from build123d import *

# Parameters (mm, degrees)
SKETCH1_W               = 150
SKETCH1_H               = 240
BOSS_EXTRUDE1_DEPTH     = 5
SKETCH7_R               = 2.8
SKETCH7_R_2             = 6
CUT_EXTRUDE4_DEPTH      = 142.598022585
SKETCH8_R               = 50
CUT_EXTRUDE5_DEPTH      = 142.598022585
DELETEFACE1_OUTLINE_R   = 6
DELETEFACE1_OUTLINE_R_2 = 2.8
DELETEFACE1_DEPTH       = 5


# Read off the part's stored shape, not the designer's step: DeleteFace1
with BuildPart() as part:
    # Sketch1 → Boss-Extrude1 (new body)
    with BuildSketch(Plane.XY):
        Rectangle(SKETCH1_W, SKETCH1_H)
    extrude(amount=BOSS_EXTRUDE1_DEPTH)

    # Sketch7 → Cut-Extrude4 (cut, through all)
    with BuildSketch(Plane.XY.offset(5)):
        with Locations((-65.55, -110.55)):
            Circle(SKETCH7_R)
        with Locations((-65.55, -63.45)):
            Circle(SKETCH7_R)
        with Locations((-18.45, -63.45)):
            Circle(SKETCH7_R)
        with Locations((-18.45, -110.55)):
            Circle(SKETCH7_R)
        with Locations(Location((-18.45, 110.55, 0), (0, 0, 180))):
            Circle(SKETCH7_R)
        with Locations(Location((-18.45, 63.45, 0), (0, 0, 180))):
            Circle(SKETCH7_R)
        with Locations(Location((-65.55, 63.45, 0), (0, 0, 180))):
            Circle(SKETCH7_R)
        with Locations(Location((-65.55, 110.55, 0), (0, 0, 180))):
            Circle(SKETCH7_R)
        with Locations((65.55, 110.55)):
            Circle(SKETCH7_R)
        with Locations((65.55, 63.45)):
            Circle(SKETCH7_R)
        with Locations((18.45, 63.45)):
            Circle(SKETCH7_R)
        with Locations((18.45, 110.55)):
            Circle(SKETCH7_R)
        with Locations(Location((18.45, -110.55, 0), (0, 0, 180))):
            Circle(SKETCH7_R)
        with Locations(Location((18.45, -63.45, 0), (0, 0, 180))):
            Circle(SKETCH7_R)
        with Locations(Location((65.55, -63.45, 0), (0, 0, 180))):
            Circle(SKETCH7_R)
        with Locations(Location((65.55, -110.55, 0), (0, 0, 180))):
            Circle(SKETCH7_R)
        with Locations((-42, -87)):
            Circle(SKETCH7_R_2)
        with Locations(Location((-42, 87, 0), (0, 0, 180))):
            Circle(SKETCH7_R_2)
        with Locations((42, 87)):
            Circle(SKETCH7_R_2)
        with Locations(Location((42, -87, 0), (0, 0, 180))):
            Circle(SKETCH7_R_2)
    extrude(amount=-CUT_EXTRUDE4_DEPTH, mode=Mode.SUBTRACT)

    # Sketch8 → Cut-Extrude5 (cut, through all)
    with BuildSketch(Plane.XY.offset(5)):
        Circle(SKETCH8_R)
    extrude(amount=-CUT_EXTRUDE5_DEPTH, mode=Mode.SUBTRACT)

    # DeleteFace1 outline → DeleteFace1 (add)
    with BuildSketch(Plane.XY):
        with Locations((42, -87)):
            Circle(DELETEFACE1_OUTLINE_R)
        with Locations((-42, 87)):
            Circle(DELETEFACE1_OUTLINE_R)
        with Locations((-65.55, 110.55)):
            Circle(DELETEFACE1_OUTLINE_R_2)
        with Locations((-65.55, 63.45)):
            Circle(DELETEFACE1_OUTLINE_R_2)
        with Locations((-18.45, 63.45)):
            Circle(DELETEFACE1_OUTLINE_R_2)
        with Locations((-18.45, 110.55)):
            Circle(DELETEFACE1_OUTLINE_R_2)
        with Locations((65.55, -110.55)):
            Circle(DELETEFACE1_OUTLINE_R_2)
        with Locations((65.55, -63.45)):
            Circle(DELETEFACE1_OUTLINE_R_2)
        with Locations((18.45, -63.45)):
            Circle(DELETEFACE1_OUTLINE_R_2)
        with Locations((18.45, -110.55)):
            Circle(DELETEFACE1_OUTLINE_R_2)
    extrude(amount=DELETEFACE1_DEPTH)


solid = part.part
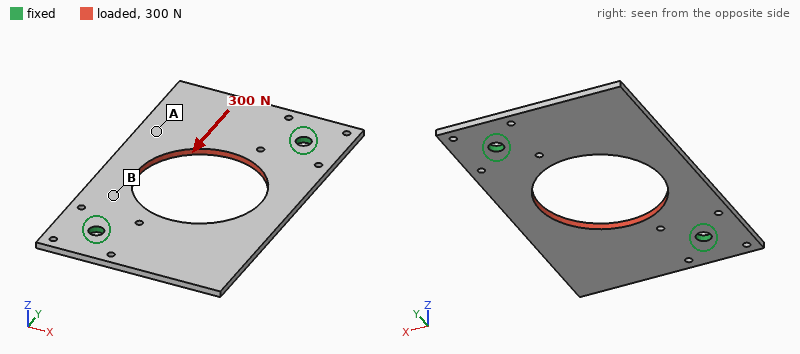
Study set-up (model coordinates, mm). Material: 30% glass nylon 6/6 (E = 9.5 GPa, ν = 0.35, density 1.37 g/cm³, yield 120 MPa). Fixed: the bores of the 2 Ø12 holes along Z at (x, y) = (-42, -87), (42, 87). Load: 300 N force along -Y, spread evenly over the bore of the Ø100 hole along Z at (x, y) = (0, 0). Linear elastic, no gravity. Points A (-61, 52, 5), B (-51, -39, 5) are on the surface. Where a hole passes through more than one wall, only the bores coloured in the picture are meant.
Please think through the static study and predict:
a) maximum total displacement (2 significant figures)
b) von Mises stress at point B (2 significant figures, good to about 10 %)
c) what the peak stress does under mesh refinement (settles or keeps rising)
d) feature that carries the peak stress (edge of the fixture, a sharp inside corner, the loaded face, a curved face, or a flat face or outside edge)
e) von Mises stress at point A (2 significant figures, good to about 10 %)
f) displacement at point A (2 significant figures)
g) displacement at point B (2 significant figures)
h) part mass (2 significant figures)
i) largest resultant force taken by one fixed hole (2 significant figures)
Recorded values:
7.1 µm
0.55 MPa
keeps rising
edge of the fixture
0.18 MPa
6.3 µm
2.9 µm
190 g
150 N
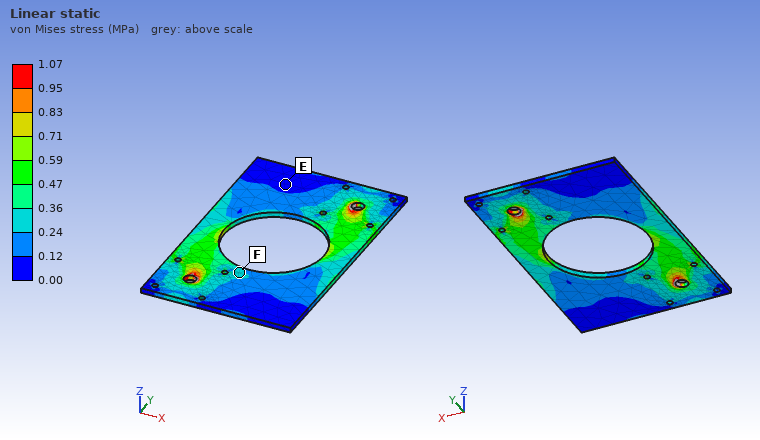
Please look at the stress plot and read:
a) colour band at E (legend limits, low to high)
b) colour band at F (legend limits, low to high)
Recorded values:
0.00 to 0.12 MPa
0.24 to 0.36 MPa
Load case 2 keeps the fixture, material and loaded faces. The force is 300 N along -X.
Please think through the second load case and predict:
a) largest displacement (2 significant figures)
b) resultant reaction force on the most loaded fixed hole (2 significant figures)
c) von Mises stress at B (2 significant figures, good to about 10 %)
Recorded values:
10 µm
150 N
0.42 MPa
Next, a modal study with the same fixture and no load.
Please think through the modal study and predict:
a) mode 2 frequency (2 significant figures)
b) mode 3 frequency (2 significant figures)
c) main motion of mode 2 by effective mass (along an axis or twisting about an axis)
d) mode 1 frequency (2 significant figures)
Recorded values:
190 Hz
410 Hz
along Z
170 Hz
